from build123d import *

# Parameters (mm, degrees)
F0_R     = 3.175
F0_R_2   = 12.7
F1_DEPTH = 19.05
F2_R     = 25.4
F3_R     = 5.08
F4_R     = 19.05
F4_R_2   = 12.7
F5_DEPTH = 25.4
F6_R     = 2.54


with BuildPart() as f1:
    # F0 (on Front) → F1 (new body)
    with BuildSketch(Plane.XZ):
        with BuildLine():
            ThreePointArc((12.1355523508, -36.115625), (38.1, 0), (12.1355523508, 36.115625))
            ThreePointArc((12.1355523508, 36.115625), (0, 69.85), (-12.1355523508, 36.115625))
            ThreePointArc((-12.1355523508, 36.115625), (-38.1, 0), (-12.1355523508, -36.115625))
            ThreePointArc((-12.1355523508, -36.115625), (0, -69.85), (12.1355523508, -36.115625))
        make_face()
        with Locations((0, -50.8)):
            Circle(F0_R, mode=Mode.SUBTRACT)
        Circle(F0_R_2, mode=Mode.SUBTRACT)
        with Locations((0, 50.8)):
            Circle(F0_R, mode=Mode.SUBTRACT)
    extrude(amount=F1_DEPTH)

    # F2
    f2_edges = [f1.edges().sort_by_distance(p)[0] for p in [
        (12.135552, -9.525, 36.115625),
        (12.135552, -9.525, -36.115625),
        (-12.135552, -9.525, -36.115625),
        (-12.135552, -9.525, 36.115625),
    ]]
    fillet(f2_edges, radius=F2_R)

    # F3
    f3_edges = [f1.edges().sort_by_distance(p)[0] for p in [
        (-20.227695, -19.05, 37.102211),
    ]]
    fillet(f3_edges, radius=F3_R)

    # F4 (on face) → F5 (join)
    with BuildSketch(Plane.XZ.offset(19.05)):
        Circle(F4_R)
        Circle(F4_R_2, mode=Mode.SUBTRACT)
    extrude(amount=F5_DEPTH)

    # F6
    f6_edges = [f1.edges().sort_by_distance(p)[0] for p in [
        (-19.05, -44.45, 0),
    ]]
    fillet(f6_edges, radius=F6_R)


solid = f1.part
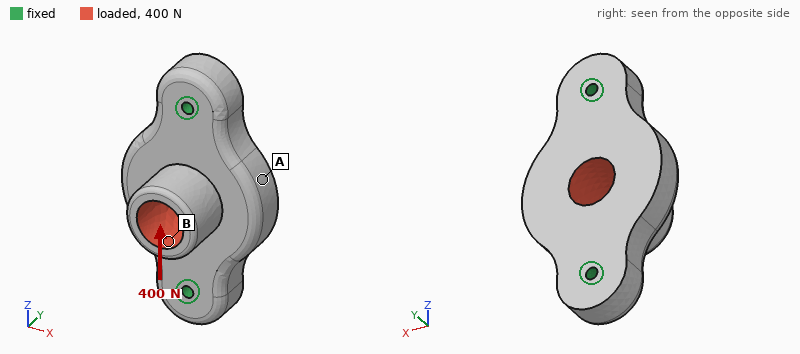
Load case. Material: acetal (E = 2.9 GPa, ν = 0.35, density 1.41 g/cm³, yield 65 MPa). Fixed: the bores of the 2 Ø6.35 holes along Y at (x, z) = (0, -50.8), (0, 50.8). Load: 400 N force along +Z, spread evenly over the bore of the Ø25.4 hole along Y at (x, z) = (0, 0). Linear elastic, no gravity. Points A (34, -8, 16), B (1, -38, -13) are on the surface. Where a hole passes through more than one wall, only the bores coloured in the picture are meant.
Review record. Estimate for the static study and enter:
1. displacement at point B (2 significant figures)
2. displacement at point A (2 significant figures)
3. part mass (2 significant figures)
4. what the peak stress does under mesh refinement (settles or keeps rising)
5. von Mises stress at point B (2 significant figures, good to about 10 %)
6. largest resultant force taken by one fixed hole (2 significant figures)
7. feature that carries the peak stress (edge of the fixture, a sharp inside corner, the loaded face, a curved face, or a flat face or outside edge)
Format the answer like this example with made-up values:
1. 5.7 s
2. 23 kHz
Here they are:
1. 22 µm
2. 4.7 µm
3. 190 g
4. keeps rising
5. 0.33 MPa
6. 210 N
7. edge of the fixture
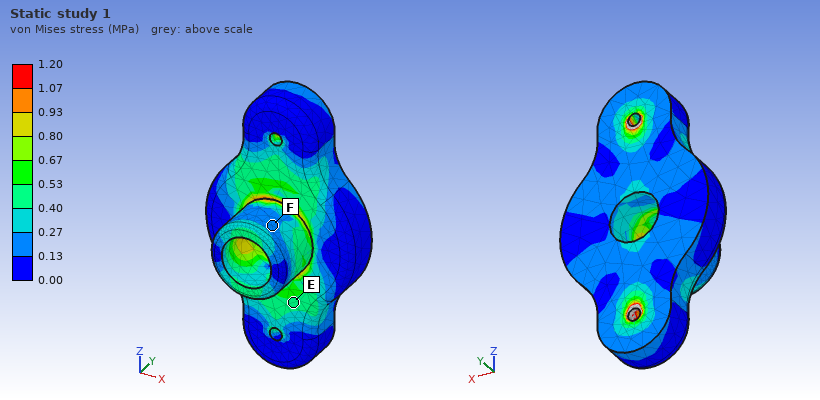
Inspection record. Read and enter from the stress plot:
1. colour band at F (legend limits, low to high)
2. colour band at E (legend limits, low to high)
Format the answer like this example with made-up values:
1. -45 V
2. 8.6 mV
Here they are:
1. 0.13 to 0.27 MPa
2. 0.40 to 0.53 MPa
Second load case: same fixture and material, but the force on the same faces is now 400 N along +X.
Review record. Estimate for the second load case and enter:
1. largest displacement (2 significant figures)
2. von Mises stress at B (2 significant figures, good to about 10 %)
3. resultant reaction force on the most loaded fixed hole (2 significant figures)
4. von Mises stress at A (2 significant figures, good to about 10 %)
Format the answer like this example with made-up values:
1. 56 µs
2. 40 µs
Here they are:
1. 76 µm
2. 0.57 MPa
3. 200 N
4. 0.45 MPa
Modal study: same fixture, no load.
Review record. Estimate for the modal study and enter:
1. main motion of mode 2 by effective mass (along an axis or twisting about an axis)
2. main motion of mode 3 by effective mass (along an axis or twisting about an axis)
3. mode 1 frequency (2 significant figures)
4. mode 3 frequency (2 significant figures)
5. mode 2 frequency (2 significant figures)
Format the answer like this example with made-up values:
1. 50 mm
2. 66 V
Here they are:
1. along Y
2. along X
3. 1300 Hz
4. 2500 Hz
5. 1500 Hz
